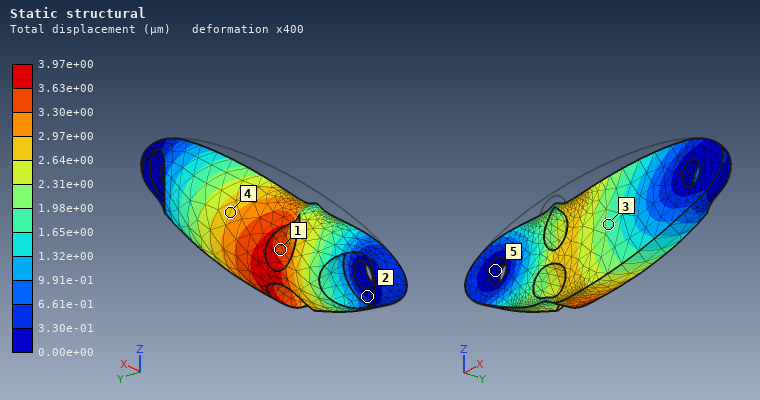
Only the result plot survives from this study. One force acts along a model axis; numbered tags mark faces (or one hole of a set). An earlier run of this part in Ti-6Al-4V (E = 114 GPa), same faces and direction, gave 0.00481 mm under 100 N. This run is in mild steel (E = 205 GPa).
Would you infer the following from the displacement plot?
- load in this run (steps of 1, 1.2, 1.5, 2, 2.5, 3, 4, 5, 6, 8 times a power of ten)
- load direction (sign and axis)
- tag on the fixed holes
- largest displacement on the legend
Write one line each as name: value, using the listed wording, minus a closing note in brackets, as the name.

load in this run: 150 N
load direction: -Z
tag on the fixed holes: 5
largest displacement on the legend: 3.97e+00 µm
